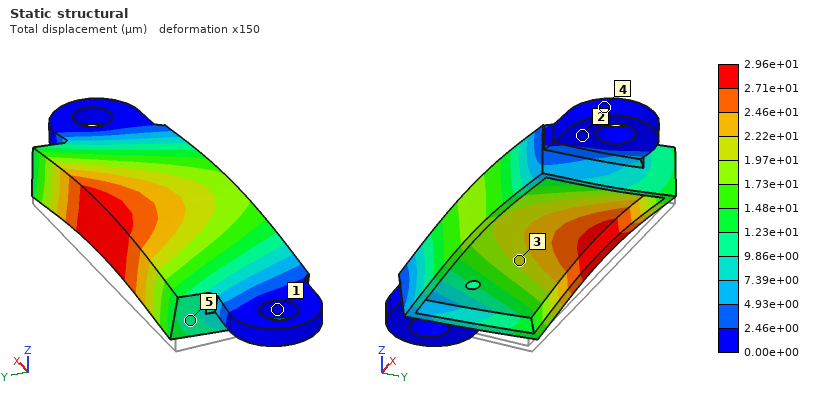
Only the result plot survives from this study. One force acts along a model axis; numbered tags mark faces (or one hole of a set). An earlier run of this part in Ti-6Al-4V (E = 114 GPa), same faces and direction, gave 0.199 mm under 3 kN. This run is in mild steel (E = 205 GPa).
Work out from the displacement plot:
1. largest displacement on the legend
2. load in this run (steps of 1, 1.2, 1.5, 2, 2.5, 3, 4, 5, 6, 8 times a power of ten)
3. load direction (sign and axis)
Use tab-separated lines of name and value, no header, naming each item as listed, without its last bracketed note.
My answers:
largest displacement on the legend	2.96e+01 µm
load in this run	800 N
load direction	+Z
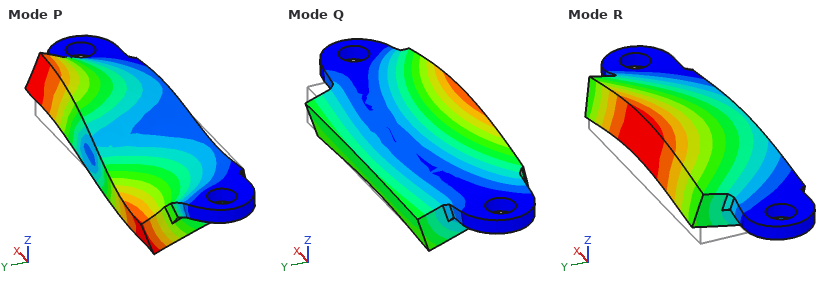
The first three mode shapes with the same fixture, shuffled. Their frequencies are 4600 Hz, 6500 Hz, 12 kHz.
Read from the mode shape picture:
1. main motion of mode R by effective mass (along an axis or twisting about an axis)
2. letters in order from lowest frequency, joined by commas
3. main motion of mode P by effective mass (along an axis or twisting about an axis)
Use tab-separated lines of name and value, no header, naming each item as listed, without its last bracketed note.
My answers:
main motion of mode R by effective mass	along Z
letters in order from lowest frequency, joined by commas	R, Q, P
main motion of mode P by effective mass	twisting about Y
